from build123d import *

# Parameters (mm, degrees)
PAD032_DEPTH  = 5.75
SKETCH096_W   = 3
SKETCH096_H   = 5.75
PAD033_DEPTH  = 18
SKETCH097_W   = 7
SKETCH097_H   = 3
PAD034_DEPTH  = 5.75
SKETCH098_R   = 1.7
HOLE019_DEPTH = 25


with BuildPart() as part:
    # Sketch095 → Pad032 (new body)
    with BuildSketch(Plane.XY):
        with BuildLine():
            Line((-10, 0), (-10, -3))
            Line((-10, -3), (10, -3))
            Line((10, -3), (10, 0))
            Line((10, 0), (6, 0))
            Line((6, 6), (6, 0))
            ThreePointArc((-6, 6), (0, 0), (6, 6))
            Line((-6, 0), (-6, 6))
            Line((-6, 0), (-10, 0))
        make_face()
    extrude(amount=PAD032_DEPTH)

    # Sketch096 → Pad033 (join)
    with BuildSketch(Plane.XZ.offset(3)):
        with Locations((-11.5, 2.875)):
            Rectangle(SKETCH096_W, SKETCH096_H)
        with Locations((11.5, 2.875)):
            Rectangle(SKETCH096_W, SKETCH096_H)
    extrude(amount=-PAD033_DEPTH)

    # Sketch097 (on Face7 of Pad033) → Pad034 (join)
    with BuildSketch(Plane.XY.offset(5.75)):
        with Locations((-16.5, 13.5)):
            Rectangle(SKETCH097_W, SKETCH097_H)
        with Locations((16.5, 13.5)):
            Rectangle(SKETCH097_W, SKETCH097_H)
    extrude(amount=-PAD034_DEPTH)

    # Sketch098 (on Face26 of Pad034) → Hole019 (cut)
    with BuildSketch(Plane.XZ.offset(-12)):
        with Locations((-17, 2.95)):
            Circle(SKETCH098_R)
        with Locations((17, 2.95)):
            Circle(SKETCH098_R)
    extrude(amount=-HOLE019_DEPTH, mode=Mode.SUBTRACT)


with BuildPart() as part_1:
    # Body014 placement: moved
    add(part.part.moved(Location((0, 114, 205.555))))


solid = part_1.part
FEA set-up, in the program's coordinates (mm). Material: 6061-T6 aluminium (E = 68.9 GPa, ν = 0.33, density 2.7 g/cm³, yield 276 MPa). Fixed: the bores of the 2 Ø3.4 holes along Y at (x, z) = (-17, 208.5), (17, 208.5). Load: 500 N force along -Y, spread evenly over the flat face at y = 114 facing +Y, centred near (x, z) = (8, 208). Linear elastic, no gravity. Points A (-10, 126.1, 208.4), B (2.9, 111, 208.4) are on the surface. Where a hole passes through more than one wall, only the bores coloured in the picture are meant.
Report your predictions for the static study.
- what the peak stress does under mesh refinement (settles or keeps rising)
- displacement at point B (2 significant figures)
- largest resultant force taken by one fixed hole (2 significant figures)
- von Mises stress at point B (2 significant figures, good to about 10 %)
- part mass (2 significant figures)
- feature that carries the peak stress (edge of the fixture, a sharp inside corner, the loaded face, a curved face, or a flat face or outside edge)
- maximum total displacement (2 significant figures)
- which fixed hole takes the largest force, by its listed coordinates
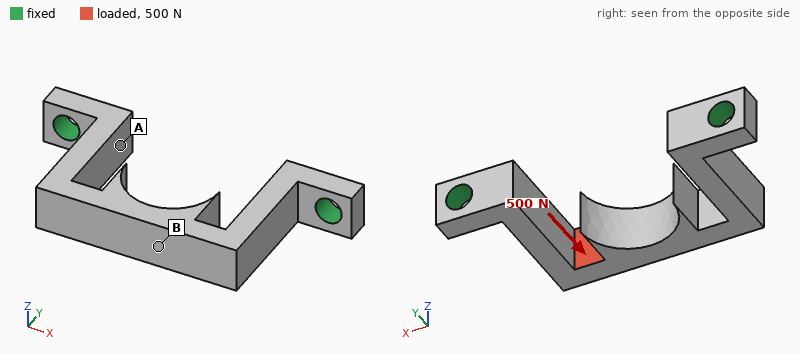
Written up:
keeps rising
35 µm
430 N
47 MPa
3.4 g
edge of the fixture
44 µm
(17, 208.5)
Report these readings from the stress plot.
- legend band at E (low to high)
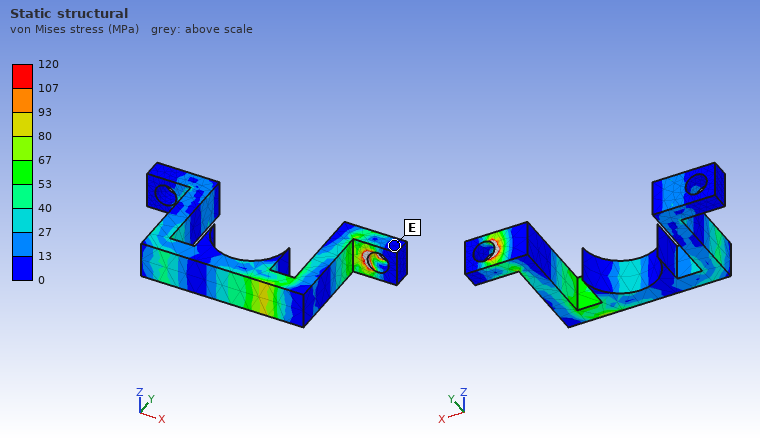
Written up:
0 to 13 MPa
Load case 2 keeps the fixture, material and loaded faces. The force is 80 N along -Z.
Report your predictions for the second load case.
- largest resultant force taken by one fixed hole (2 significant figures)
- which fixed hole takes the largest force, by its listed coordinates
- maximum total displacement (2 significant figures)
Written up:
62 N
(17, 208.5)
59 µm
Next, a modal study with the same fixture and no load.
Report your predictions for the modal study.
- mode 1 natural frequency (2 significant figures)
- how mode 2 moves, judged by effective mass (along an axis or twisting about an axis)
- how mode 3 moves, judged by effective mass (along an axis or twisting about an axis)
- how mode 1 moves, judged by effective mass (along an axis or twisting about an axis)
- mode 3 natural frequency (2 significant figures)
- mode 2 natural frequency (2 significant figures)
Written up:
5200 Hz
along X
twisting about Y
along Z
10 kHz
6600 Hz
